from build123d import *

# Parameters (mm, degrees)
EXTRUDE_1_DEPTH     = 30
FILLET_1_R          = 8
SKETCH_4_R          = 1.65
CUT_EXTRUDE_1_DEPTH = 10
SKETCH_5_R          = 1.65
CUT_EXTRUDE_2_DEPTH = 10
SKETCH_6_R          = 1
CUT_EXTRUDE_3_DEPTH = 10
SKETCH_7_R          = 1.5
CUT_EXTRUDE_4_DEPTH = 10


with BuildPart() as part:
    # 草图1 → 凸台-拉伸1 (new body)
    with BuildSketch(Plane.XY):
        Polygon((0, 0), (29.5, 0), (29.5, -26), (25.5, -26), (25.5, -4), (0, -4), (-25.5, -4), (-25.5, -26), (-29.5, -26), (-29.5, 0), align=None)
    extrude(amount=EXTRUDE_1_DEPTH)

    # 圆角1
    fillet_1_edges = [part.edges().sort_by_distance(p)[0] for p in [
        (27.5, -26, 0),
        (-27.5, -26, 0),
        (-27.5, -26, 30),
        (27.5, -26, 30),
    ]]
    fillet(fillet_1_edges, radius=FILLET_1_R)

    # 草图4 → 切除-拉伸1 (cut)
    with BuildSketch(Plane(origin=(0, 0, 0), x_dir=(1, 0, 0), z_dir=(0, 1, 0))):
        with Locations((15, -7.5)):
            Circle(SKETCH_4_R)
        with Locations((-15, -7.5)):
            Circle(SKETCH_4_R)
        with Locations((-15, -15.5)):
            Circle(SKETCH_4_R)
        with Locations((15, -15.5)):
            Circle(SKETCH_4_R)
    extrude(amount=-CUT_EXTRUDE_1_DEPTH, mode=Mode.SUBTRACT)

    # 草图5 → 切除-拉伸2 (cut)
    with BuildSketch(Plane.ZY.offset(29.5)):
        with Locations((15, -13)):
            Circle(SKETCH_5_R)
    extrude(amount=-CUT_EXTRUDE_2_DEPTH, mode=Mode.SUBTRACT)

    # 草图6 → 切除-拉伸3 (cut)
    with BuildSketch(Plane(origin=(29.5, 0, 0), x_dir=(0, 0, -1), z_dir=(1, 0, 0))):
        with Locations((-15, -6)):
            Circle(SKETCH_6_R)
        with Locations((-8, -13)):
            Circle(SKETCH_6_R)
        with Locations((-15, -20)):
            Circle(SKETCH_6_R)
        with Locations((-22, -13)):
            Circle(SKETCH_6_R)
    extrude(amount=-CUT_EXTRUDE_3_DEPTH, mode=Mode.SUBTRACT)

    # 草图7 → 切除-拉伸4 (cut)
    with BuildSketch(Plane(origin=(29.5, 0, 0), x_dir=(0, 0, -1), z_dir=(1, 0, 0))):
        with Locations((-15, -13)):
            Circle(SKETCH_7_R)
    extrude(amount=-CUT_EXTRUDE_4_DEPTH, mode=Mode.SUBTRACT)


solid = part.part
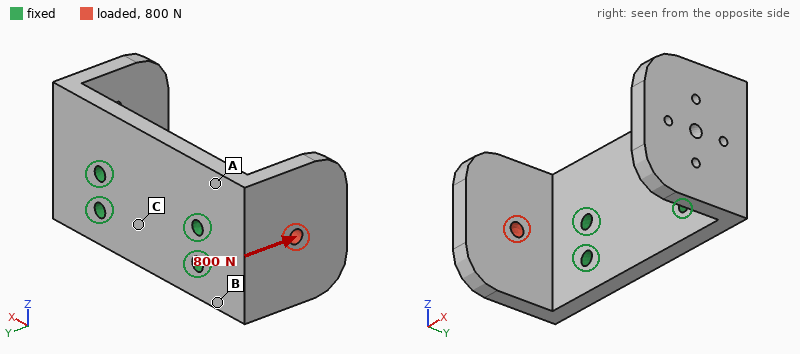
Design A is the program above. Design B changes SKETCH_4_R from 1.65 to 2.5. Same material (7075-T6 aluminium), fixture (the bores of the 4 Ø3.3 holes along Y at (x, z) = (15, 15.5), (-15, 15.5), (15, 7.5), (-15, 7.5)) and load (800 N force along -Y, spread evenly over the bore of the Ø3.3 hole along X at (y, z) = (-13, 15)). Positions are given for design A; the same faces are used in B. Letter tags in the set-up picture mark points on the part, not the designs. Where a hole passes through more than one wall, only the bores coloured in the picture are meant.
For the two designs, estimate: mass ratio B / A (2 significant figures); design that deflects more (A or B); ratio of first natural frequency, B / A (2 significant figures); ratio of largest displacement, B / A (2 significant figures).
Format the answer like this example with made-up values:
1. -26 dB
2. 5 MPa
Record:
1. 0.99
2. A
3. 1.1
4. 0.82
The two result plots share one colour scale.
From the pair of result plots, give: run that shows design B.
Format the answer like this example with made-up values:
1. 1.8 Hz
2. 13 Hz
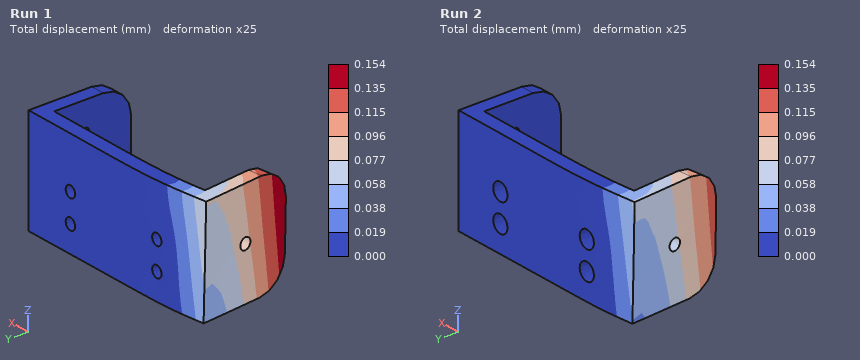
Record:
1. Run 2
